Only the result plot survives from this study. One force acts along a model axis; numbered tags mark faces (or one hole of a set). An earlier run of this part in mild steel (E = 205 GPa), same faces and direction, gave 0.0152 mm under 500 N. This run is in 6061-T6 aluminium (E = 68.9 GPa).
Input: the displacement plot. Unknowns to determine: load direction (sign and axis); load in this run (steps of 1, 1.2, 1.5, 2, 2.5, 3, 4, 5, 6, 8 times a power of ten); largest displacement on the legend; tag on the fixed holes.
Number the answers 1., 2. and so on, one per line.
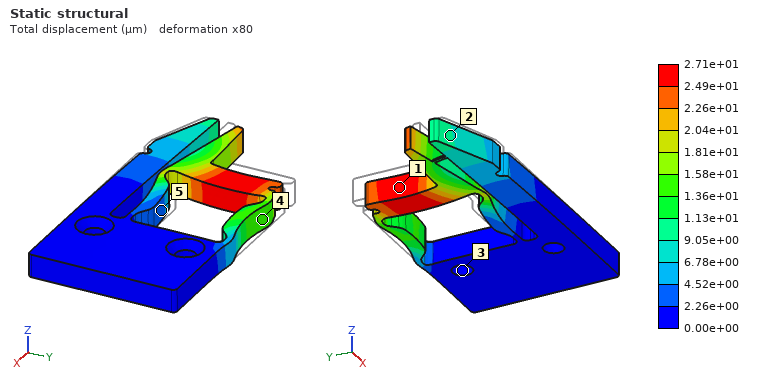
1. +X
2. 300 N
3. 2.71e+01 µm
4. 3
